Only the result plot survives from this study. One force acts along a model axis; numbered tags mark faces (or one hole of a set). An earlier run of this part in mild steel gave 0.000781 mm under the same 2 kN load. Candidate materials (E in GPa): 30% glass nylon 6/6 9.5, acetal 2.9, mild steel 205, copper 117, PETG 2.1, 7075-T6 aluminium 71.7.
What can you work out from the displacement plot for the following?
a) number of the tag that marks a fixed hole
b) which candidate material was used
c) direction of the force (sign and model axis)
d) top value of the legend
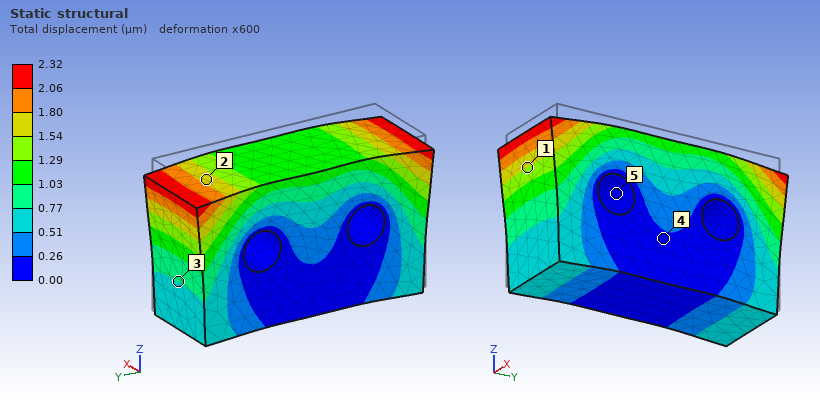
5
7075-T6 aluminium
-Z
2.32 µm
